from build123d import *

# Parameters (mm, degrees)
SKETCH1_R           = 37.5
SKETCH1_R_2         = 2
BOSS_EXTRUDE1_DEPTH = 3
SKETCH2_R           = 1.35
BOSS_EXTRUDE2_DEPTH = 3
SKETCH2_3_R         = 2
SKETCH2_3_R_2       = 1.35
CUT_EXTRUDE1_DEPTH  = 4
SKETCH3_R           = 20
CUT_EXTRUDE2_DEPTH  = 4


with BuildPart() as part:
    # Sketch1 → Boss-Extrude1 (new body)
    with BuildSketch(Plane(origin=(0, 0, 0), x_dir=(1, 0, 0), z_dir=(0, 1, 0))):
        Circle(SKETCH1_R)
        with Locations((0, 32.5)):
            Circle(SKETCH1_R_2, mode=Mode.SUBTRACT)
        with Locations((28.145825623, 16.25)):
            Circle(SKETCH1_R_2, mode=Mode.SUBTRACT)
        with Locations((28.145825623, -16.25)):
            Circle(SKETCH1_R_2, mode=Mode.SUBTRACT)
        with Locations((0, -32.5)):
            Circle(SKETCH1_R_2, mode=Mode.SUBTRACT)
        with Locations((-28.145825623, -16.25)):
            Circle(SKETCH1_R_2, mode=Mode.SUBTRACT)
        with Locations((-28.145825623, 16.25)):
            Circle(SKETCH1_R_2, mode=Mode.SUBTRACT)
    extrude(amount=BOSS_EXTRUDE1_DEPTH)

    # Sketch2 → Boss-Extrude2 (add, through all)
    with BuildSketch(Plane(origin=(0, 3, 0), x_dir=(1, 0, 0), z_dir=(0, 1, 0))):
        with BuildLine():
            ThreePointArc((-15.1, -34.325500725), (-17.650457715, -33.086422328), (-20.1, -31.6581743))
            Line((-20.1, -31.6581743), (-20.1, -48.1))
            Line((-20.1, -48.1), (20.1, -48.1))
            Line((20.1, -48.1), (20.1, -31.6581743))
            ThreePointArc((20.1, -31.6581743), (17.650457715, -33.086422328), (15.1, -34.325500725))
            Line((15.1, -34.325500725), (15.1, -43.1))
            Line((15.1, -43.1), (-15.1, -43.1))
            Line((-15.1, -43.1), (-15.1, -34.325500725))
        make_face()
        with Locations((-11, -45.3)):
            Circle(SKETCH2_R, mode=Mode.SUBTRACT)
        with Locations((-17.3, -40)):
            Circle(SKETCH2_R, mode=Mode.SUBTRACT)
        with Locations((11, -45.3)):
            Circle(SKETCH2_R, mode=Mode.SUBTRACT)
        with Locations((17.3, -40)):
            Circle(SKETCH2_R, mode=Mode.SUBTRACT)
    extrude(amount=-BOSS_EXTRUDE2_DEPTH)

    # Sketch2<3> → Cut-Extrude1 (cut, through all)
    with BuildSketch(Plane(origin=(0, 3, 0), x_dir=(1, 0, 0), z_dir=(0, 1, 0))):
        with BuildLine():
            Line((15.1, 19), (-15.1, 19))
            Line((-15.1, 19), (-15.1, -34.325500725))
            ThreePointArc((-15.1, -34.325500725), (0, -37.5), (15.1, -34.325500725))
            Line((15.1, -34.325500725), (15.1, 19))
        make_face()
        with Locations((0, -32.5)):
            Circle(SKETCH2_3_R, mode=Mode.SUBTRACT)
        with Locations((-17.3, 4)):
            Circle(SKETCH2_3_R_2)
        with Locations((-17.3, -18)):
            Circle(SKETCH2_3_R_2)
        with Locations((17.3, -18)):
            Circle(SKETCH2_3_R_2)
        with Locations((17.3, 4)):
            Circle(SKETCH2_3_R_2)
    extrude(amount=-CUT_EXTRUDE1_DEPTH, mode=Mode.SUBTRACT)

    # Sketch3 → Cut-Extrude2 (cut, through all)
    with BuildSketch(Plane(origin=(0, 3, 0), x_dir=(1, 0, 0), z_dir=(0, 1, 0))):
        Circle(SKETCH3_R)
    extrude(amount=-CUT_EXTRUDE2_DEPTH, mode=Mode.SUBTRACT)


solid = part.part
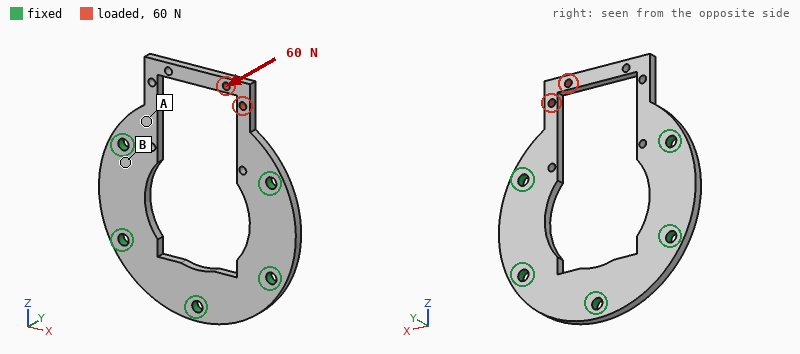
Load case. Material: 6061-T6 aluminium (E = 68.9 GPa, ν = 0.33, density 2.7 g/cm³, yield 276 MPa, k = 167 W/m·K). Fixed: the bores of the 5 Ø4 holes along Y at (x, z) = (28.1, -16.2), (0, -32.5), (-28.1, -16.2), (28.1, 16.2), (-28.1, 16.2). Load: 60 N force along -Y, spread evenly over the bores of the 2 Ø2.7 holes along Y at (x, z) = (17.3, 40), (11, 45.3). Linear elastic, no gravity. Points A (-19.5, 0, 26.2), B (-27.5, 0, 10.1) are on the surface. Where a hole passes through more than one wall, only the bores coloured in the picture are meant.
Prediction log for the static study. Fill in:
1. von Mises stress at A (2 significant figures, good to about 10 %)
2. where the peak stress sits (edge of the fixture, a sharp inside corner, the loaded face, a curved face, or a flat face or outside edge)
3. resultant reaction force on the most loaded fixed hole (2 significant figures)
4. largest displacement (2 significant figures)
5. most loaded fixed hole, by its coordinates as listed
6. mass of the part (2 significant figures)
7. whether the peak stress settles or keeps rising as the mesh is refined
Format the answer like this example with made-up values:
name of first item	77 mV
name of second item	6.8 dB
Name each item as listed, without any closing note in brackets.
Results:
von Mises stress at A	23 MPa
where the peak stress sits	edge of the fixture
resultant reaction force on the most loaded fixed hole	56 N
largest displacement	0.25 mm
most loaded fixed hole, by its coordinates as listed	(28.1, 16.2)
mass of the part	22 g
whether the peak stress settles or keeps rising as the mesh is refined	keeps rising
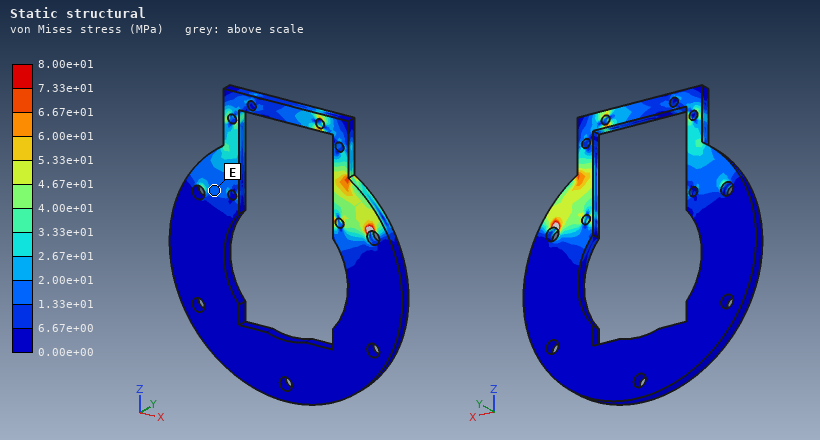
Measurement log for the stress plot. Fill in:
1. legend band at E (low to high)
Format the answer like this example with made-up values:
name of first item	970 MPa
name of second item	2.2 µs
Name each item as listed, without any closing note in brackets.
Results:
legend band at E	1.33e+01 to 2.00e+01 MPa
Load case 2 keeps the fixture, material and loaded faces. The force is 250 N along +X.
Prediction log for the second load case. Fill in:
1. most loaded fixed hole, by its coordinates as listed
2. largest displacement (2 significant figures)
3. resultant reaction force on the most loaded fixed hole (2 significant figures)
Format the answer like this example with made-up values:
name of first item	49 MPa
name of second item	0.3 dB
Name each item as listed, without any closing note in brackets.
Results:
most loaded fixed hole, by its coordinates as listed	(28.1, 16.2)
largest displacement	56 µm
resultant reaction force on the most loaded fixed hole	230 N
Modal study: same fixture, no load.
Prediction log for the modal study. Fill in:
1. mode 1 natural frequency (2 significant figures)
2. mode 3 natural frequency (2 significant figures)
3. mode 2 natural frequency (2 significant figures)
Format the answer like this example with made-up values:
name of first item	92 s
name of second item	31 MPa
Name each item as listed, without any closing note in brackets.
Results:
mode 1 natural frequency	2000 Hz
mode 3 natural frequency	7500 Hz
mode 2 natural frequency	4000 Hz
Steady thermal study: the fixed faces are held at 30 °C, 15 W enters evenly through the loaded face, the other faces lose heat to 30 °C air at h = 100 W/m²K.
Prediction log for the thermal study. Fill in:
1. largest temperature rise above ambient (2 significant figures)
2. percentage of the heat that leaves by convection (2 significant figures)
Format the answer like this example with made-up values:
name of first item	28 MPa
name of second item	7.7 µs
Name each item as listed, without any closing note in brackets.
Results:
largest temperature rise above ambient	71 K
percentage of the heat that leaves by convection	34 %
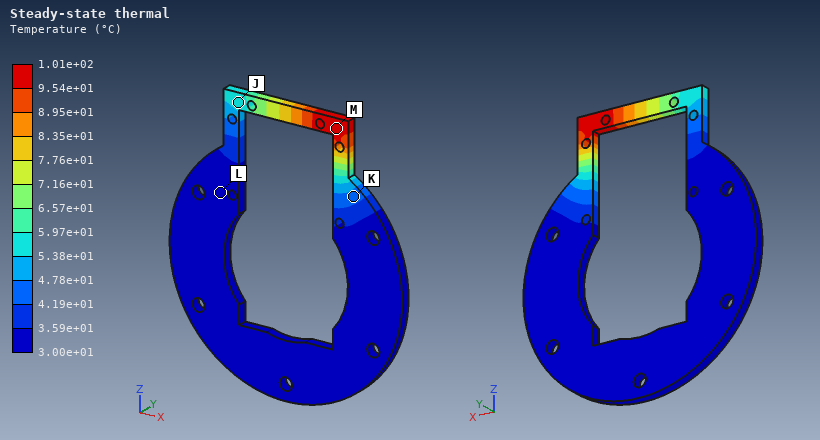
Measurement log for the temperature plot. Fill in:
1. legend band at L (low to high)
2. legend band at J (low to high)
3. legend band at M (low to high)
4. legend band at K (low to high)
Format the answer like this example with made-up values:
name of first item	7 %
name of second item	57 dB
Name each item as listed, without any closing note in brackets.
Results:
legend band at L	3.00e+01 to 3.59e+01 °C
legend band at J	5.38e+01 to 5.97e+01 °C
legend band at M	9.54e+01 to 1.01e+02 °C
legend band at K	4.19e+01 to 4.78e+01 °C
